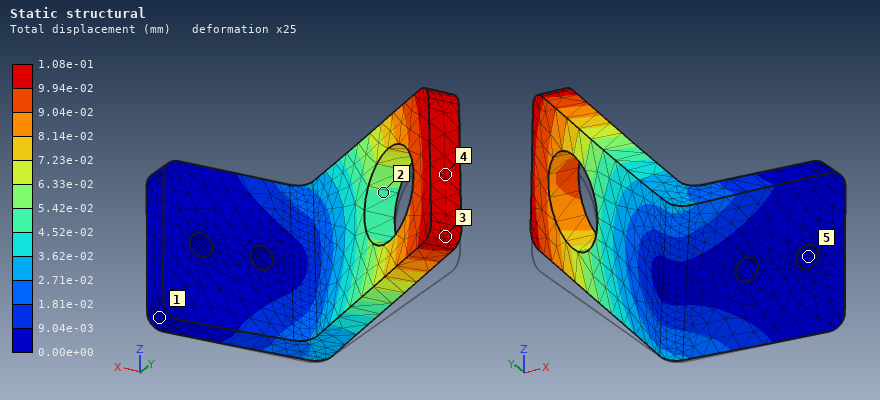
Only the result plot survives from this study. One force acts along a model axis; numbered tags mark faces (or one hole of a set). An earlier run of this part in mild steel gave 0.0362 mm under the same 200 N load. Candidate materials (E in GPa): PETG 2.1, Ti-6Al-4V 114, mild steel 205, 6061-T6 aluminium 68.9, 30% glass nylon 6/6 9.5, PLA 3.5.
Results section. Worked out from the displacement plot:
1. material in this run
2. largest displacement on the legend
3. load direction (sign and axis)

6061-T6 aluminium
1.08e-01 mm
+Z
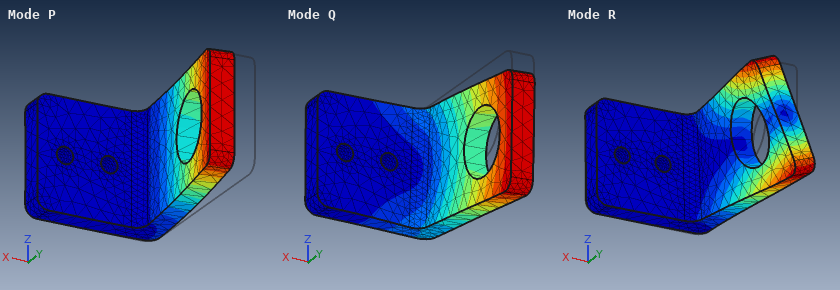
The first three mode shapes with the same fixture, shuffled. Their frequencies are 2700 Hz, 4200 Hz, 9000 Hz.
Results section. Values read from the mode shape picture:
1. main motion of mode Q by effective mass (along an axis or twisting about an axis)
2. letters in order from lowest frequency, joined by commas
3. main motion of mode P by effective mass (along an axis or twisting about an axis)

along Z
P, Q, R
along X
